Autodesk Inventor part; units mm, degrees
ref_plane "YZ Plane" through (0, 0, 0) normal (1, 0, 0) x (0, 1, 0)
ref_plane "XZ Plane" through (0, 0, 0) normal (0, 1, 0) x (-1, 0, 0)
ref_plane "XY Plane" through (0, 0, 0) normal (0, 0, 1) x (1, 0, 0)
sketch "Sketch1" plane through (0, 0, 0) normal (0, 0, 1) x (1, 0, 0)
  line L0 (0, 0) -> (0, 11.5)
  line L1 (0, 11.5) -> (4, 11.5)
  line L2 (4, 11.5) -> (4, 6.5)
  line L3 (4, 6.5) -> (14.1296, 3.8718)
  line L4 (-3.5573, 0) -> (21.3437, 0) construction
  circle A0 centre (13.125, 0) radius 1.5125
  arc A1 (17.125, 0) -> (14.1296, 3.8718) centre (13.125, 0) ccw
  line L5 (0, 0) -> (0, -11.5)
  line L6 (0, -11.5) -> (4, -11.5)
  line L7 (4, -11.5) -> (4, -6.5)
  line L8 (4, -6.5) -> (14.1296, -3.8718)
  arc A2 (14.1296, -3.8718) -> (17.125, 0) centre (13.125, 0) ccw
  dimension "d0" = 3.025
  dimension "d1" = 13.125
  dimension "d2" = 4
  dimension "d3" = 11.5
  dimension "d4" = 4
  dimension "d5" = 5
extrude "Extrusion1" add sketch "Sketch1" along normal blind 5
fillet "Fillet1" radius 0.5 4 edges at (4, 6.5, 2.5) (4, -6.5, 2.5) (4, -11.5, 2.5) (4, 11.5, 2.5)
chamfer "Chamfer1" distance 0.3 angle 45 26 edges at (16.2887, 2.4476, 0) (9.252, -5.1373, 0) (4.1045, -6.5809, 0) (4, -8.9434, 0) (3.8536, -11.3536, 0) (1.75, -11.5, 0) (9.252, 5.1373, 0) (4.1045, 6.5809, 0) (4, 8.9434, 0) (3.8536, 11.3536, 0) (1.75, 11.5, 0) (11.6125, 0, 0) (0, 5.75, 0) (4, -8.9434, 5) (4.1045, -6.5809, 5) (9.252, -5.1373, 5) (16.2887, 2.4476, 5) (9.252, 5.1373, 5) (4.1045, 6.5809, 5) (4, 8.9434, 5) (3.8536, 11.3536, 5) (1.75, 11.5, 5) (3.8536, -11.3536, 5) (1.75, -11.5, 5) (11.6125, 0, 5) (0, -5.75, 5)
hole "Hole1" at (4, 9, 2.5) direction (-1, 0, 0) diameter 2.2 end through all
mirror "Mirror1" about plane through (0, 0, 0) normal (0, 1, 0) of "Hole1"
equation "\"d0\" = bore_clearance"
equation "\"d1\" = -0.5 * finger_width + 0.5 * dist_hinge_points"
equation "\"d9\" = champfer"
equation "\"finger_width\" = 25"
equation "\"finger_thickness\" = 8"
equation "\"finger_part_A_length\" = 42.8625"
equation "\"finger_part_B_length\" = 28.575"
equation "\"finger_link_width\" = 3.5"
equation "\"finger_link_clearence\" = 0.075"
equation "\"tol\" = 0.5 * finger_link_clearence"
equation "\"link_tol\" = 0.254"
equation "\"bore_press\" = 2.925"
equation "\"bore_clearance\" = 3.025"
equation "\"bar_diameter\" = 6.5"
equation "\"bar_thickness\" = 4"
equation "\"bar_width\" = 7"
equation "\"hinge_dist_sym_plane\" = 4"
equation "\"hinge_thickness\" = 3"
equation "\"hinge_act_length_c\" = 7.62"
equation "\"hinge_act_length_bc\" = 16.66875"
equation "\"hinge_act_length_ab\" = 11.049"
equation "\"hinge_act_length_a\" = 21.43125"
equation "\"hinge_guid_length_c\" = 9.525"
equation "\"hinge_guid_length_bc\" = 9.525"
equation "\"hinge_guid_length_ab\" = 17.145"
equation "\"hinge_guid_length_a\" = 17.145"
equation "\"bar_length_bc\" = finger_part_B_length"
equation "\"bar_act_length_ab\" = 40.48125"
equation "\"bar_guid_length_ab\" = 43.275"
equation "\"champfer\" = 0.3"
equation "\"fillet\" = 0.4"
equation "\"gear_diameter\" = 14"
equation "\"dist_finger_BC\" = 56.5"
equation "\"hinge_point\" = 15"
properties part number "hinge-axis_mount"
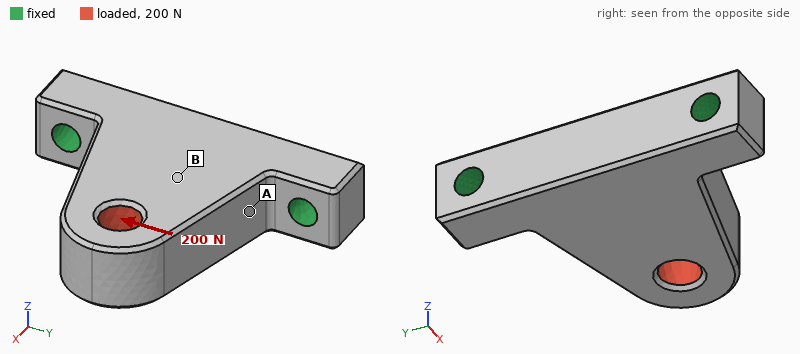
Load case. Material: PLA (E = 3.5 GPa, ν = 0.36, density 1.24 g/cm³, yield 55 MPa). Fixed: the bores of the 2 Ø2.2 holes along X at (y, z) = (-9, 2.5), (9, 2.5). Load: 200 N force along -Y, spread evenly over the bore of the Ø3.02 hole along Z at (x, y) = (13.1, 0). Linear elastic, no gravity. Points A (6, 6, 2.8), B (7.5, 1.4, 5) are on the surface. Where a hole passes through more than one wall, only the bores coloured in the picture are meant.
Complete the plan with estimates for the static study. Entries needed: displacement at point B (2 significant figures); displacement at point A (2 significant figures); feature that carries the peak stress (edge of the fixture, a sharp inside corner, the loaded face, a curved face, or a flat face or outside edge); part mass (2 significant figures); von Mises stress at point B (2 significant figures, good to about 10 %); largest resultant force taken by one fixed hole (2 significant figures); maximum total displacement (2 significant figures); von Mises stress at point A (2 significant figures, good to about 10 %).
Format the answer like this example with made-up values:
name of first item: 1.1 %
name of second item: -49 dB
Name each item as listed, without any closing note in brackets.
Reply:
displacement at point B: 0.033 mm
displacement at point A: 0.035 mm
feature that carries the peak stress: a curved face
part mass: 1.2 g
von Mises stress at point B: 6.7 MPa
largest resultant force taken by one fixed hole: 180 N
maximum total displacement: 0.13 mm
von Mises stress at point A: 17 MPa
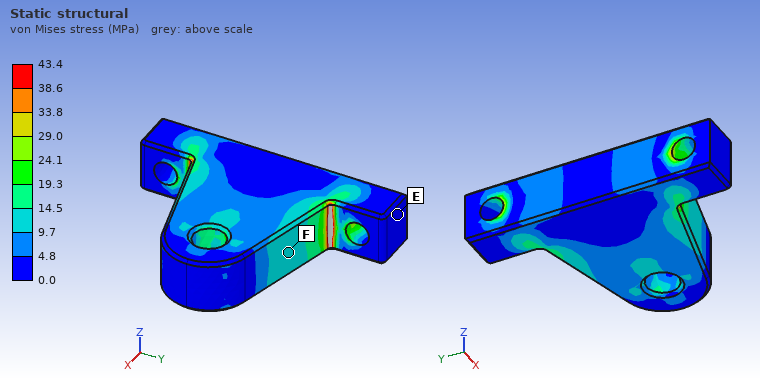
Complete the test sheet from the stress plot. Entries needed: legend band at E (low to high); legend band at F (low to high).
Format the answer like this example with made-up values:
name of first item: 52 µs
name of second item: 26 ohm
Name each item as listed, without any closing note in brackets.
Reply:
legend band at E: 0.0 to 4.8 MPa
legend band at F: 9.7 to 14.5 MPa
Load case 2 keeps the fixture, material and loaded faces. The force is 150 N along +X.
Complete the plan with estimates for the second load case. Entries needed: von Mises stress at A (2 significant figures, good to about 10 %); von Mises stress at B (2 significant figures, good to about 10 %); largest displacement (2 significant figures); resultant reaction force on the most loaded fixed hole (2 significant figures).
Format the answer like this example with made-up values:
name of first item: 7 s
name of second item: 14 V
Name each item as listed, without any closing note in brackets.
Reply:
von Mises stress at A: 6.3 MPa
von Mises stress at B: 2.1 MPa
largest displacement: 29 µm
resultant reaction force on the most loaded fixed hole: 82 N
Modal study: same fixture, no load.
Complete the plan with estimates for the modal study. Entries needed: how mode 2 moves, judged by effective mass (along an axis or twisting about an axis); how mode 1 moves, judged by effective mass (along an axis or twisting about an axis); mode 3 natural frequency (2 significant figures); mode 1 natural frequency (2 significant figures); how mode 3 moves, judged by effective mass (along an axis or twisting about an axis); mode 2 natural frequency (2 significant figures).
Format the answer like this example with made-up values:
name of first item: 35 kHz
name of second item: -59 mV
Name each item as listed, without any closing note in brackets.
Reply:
how mode 2 moves, judged by effective mass: along Y
how mode 1 moves, judged by effective mass: along Z
mode 3 natural frequency: 14 kHz
mode 1 natural frequency: 4000 Hz
how mode 3 moves, judged by effective mass: along X
mode 2 natural frequency: 12 kHz
